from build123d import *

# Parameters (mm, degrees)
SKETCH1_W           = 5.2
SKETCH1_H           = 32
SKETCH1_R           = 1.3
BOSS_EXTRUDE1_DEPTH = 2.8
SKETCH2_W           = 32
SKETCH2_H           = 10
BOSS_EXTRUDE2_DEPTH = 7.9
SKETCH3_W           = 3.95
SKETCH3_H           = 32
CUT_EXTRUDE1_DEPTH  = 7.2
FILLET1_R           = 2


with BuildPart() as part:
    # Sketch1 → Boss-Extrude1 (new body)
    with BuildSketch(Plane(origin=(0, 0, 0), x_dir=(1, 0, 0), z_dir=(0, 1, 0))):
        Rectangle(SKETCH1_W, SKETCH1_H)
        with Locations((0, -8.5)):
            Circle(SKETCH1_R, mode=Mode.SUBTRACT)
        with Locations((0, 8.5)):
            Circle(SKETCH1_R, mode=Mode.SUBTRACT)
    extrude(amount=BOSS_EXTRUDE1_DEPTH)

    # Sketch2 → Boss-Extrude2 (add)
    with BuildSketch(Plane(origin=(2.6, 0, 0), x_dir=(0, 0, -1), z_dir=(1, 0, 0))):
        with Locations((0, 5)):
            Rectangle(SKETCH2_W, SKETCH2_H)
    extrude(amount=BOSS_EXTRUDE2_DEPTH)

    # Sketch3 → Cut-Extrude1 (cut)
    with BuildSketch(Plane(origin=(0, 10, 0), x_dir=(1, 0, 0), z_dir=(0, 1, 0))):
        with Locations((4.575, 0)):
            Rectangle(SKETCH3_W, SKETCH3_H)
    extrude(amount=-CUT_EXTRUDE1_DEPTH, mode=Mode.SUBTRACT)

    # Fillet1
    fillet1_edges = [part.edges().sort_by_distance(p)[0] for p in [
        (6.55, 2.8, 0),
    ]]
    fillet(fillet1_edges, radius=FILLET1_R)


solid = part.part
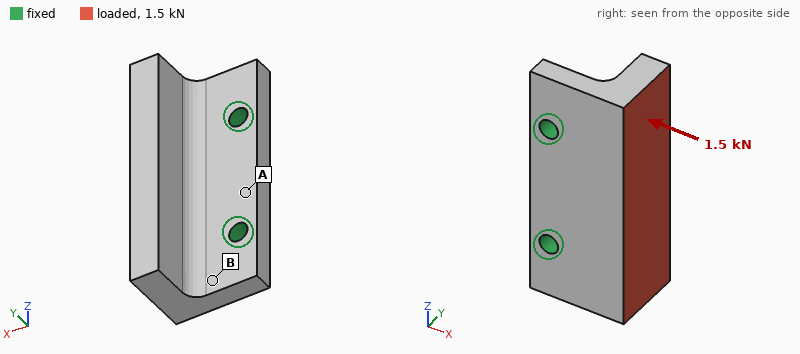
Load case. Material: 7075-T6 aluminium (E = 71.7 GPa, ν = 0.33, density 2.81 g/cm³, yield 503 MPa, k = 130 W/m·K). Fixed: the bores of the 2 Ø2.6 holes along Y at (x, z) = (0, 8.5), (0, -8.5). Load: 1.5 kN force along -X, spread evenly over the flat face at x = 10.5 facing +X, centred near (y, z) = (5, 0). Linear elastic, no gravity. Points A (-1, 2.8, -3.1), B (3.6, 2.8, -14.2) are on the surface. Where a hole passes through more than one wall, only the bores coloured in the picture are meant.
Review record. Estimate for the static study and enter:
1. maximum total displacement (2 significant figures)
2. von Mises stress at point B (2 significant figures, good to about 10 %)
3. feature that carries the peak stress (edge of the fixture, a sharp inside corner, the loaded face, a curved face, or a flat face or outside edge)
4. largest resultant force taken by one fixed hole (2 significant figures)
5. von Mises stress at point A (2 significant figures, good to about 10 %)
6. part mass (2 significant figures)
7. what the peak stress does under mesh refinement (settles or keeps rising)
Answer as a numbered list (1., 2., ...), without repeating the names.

1. 0.11 mm
2. 110 MPa
3. edge of the fixture
4. 750 N
5. 51 MPa
6. 5.8 g
7. keeps rising
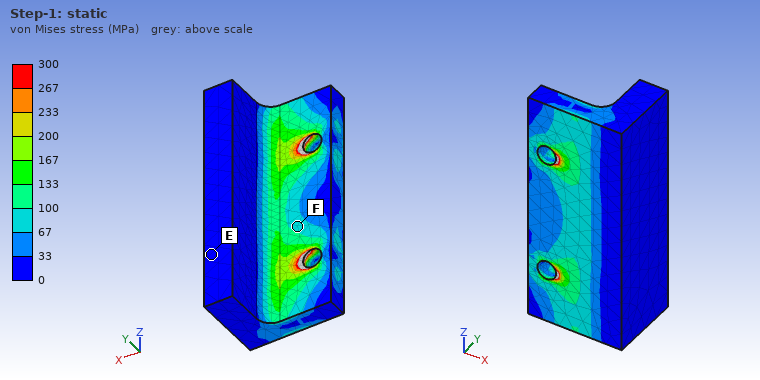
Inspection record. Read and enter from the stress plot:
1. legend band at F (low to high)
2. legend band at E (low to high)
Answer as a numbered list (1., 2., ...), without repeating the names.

1. 67 to 100 MPa
2. 0 to 33 MPa
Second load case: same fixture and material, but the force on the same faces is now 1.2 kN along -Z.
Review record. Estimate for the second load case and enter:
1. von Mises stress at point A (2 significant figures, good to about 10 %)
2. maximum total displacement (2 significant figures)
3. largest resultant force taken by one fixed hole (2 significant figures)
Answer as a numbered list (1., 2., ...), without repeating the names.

1. 16 MPa
2. 23 µm
3. 900 N
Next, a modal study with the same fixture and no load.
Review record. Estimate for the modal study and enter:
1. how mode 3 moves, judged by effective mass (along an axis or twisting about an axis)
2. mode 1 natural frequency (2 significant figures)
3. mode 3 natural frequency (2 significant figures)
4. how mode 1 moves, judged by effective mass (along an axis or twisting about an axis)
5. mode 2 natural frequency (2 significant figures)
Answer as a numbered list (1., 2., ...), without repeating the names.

1. along Z
2. 8200 Hz
3. 26 kHz
4. along Y
5. 14 kHz
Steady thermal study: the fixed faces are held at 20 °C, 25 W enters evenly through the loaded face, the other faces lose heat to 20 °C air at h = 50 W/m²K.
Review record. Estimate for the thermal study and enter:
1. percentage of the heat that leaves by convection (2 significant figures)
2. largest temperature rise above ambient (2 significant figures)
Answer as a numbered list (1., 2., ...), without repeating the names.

1. 3.5 %
2. 24 K
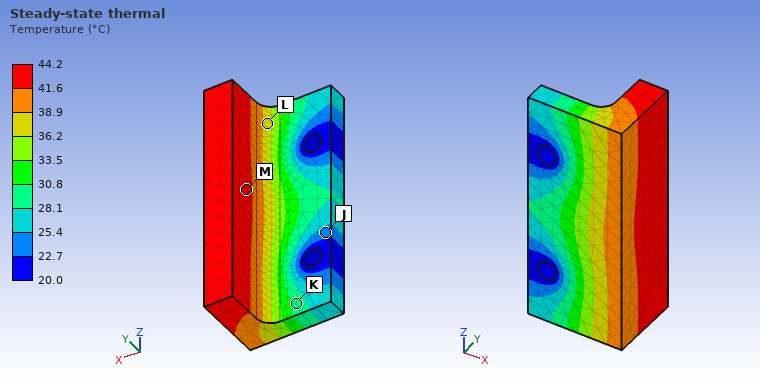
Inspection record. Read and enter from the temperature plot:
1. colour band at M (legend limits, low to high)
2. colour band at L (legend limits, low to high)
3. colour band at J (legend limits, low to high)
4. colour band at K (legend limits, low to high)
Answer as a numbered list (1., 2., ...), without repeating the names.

1. 41.6 to 44.2 °C
2. 36.2 to 38.9 °C
3. 22.7 to 25.4 °C
4. 28.1 to 30.8 °C
